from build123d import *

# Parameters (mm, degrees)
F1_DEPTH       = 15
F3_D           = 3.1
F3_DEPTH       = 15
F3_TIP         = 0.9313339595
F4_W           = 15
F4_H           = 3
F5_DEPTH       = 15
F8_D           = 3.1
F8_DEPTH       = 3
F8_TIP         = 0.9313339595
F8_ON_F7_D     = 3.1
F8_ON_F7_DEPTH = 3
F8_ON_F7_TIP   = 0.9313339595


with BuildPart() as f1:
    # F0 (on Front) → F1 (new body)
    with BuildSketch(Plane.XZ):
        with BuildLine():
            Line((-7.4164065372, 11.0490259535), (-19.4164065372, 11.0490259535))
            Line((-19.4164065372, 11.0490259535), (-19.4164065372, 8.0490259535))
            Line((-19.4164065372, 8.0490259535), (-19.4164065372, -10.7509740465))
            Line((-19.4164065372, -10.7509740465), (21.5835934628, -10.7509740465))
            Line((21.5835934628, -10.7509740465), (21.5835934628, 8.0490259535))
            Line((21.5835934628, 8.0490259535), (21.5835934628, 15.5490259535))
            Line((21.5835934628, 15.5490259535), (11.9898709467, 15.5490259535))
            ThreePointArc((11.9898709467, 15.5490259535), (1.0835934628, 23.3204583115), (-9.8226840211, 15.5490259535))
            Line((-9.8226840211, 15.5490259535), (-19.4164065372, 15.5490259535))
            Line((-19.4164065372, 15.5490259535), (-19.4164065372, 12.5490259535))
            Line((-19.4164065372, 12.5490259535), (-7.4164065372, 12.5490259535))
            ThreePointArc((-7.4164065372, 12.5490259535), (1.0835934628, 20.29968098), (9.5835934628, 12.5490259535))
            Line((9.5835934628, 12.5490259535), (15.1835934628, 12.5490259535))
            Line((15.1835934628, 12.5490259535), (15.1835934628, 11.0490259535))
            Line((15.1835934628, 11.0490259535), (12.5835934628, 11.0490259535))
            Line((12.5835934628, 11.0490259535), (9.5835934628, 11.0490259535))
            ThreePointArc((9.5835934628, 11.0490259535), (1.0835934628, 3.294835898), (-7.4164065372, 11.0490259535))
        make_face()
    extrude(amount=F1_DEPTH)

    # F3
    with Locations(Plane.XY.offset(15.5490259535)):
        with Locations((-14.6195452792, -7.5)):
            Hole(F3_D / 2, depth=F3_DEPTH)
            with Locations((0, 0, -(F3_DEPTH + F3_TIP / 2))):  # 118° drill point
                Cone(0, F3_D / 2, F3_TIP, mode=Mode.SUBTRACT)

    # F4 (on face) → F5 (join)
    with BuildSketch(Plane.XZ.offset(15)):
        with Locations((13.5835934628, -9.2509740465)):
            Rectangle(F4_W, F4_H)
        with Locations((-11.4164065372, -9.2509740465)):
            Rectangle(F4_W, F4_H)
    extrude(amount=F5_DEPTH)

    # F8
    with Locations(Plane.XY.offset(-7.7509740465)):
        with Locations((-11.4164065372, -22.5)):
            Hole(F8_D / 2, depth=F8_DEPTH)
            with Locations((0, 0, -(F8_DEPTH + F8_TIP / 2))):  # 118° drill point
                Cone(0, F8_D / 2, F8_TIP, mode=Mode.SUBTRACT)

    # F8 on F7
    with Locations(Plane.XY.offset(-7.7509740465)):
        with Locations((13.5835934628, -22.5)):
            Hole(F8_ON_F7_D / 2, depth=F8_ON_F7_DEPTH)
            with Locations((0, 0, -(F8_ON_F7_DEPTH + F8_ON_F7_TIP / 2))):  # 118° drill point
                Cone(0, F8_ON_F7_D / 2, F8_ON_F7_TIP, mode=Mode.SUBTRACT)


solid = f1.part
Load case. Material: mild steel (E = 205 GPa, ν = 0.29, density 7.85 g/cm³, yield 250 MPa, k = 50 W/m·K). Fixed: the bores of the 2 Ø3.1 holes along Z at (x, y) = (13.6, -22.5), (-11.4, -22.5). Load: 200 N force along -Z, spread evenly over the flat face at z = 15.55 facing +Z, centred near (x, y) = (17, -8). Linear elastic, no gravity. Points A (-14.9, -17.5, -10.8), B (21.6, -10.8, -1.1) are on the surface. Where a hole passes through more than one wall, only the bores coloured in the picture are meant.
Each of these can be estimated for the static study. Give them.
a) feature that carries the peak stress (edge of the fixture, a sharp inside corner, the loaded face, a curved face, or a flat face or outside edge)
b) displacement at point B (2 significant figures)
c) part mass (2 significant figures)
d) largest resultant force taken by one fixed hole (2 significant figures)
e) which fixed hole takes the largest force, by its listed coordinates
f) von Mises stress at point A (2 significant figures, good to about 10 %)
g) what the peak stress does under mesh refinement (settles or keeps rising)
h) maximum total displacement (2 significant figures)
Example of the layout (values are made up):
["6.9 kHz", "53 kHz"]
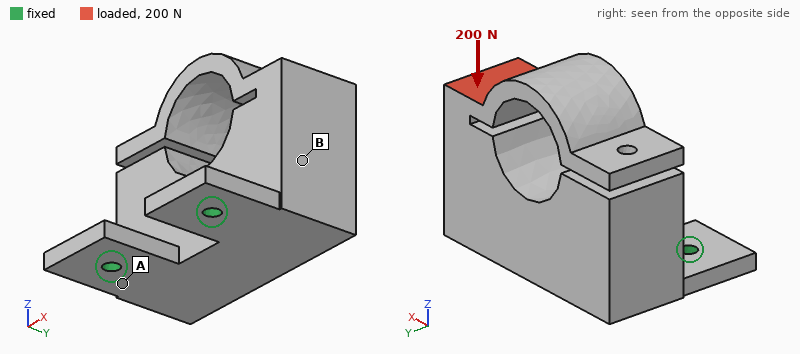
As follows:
["edge of the fixture", "18 µm", "120 g", "210 N", "(13.6, -22.5)", "42 MPa", "keeps rising", "51 µm"]
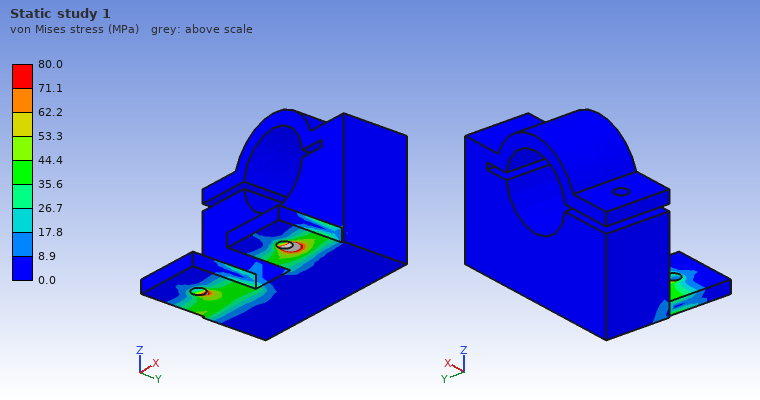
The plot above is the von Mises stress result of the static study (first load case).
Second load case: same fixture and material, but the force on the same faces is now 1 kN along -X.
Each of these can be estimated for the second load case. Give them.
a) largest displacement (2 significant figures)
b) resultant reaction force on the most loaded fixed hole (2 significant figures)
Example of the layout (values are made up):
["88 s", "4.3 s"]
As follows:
["65 µm", "1.2 kN"]
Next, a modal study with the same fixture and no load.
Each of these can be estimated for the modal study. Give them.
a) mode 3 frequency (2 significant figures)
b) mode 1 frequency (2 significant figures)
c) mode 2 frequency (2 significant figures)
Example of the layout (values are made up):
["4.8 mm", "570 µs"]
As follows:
["3300 Hz", "1000 Hz", "1700 Hz"]
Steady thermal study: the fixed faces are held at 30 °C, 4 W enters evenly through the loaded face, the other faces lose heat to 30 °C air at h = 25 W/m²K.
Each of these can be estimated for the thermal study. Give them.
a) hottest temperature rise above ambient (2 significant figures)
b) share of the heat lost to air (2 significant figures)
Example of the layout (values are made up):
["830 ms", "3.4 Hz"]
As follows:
["17 K", "32 %"]
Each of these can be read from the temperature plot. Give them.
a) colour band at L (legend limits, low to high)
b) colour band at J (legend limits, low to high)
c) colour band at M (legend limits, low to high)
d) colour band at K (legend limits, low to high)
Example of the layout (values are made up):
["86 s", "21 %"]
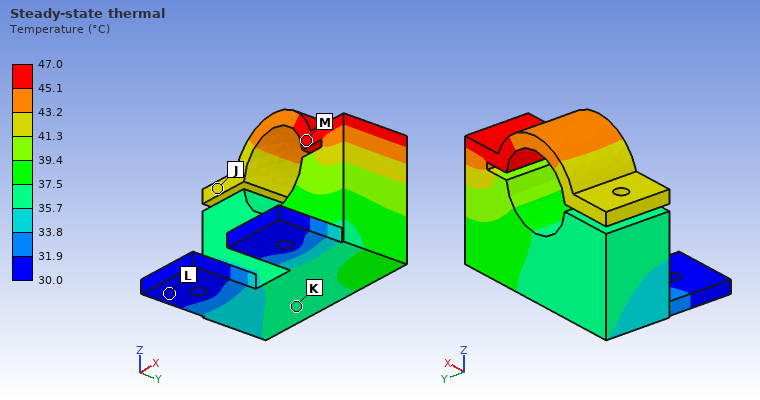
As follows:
["30.0 to 31.9 °C", "41.3 to 43.2 °C", "45.1 to 47.0 °C", "35.7 to 37.5 °C"]
